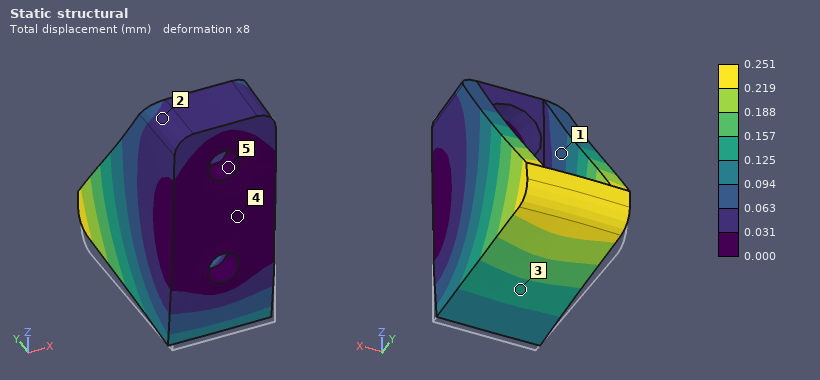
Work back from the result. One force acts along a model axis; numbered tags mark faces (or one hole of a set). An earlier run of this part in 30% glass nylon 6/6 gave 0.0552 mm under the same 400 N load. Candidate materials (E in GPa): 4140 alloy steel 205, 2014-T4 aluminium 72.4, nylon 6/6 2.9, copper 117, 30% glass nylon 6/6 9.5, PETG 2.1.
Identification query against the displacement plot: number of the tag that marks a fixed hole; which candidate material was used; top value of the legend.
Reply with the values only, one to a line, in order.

5
PETG
0.251 mm
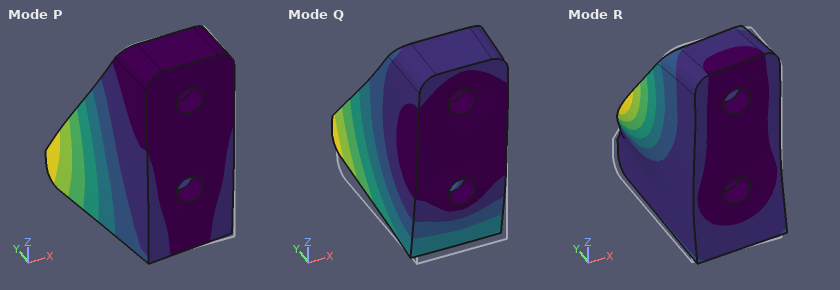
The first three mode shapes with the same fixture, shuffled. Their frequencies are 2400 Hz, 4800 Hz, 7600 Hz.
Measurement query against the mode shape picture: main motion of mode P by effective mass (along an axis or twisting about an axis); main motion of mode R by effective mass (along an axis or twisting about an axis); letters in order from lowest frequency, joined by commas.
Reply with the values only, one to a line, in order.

along X
twisting about Y
P, Q, R
